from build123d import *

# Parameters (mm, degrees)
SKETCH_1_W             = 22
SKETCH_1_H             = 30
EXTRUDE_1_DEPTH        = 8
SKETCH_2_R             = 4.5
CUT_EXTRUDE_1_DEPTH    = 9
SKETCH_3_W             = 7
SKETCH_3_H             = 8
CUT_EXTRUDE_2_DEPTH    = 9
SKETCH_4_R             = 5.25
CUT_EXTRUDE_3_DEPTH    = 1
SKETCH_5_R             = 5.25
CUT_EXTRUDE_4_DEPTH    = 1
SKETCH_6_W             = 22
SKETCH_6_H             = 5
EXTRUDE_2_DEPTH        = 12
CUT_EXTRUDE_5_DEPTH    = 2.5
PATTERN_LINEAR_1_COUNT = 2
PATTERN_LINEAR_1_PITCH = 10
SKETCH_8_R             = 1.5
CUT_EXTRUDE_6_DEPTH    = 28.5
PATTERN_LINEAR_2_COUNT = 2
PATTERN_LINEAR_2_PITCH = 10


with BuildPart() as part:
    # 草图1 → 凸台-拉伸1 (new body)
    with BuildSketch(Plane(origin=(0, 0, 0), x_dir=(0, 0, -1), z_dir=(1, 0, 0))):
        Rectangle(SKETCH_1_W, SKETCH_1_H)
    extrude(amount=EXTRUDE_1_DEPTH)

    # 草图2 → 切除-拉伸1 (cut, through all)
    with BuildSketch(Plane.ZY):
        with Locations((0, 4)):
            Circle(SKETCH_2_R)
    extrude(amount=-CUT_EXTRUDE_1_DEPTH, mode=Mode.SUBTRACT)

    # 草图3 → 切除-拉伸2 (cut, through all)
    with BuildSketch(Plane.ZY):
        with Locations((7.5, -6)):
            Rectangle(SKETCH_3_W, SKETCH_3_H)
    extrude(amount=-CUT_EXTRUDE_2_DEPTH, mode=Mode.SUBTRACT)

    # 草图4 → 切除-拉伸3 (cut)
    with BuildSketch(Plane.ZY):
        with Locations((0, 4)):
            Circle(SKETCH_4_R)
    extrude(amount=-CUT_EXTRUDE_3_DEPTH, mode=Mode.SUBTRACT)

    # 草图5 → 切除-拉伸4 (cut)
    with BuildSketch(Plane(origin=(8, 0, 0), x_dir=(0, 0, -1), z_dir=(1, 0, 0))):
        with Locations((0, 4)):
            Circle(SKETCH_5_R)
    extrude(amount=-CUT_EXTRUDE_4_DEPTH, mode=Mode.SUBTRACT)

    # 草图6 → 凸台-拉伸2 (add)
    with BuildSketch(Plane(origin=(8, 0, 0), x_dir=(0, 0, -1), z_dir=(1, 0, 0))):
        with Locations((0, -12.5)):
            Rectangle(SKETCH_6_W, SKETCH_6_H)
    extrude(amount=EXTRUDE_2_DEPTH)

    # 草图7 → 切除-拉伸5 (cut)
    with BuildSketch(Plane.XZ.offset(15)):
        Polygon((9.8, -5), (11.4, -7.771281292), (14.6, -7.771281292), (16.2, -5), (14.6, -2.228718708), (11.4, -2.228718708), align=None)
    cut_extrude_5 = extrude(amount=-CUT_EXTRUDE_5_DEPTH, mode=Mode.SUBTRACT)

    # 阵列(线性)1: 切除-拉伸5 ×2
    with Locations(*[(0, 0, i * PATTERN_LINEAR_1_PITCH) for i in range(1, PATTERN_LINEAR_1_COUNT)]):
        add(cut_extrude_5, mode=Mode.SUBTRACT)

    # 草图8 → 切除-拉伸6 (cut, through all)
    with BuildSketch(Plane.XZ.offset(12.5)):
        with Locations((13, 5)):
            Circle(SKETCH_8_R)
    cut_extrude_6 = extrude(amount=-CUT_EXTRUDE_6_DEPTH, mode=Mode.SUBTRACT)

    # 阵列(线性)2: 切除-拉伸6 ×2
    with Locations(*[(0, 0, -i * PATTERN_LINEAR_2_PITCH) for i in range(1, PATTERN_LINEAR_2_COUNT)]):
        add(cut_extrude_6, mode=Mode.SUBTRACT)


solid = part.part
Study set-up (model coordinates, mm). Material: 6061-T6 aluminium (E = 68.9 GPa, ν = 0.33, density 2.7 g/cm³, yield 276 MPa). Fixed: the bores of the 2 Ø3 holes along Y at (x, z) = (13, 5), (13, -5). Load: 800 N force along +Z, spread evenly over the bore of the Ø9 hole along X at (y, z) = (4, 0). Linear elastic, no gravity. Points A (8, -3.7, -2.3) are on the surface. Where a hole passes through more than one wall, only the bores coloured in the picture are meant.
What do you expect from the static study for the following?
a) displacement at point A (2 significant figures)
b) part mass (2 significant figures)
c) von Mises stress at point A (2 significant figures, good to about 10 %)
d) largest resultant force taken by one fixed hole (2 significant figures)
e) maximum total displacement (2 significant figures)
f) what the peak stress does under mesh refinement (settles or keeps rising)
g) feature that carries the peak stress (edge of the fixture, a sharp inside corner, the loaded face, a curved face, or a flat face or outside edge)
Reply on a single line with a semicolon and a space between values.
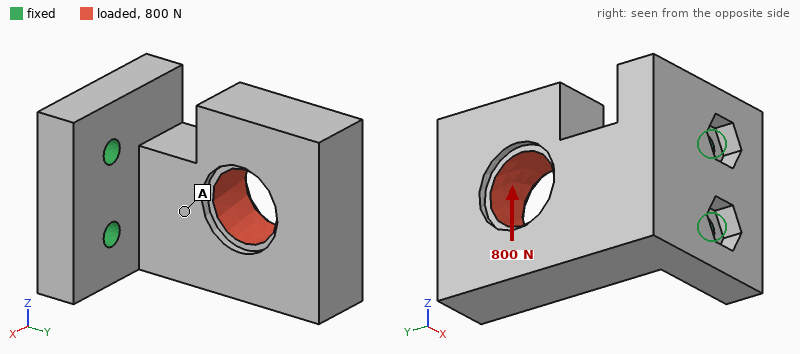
0.038 mm; 15 g; 38 MPa; 1.2 kN; 0.14 mm; keeps rising; edge of the fixture
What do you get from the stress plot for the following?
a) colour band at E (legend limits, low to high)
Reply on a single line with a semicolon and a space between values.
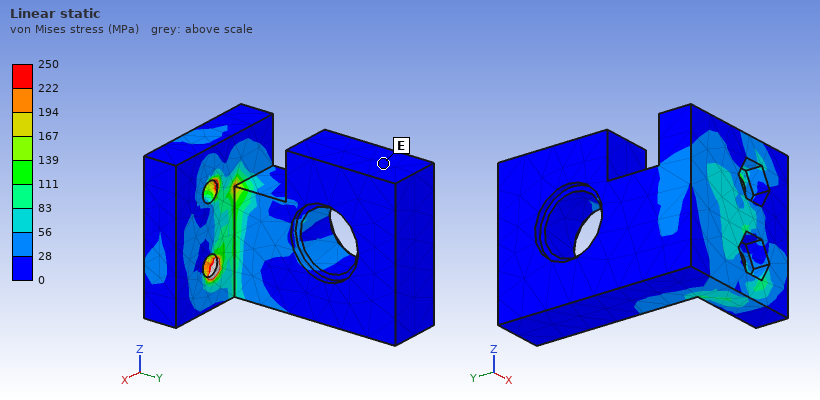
0 to 28 MPa
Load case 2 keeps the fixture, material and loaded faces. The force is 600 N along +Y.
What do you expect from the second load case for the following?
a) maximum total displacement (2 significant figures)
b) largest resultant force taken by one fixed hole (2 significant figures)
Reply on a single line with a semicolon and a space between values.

0.11 mm; 300 N
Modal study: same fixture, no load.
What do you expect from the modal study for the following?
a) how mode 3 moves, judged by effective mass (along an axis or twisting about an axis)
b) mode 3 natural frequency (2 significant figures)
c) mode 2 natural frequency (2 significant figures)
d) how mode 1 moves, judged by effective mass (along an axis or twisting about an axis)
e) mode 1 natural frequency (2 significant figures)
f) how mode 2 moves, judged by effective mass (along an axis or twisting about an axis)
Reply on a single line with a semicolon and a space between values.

along Y; 11 kHz; 4800 Hz; along X; 2700 Hz; along Z
